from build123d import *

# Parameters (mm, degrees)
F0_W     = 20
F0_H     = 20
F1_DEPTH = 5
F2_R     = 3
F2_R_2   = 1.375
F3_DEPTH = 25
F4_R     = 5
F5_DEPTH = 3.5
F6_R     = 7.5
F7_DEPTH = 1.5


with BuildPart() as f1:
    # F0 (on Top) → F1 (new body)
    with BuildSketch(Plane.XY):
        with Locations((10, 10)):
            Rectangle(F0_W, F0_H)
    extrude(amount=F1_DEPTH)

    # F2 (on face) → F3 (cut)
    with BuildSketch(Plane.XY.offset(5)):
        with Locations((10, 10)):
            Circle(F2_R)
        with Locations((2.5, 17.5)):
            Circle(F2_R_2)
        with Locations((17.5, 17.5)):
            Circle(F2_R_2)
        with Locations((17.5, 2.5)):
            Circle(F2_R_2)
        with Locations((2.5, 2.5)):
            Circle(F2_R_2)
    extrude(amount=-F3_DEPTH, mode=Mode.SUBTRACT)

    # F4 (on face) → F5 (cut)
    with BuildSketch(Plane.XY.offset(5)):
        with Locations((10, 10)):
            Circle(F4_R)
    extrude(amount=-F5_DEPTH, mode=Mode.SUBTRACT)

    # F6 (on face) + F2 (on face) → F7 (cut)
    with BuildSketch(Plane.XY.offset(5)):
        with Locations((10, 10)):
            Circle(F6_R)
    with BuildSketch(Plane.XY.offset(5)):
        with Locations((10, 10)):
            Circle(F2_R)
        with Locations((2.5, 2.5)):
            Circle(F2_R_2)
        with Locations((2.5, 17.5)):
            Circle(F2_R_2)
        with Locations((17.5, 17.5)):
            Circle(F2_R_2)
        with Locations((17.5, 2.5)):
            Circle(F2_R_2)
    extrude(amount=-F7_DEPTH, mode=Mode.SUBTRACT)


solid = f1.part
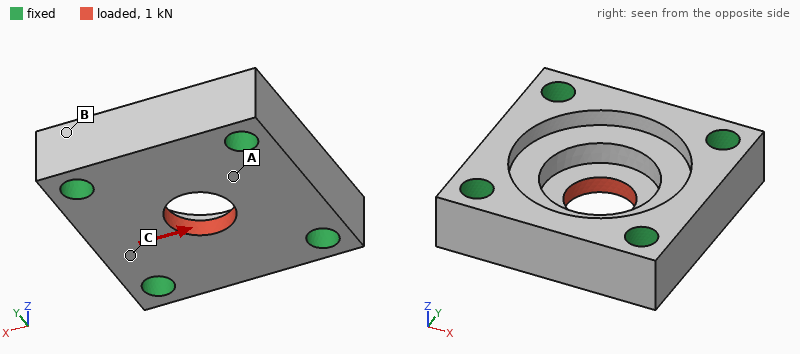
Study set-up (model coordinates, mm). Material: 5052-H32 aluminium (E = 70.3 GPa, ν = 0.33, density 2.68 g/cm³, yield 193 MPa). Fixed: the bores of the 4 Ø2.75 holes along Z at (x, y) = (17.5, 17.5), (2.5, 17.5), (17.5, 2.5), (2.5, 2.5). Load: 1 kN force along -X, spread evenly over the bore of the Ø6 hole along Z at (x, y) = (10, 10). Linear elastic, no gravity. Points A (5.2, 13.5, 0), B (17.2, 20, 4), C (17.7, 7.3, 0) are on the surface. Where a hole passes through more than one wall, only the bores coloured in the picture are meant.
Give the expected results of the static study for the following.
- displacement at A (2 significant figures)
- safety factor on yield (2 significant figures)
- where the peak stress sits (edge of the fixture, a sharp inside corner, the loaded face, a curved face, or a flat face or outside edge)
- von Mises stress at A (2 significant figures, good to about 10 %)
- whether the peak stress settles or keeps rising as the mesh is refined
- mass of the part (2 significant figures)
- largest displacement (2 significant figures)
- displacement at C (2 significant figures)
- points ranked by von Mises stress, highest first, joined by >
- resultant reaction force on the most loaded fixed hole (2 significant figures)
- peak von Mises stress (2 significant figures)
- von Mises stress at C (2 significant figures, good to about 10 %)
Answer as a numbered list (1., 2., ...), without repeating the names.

1. 1.7 µm
2. 3.0
3. the loaded face
4. 29 MPa
5. settles
6. 3.8 g
7. 4.1 µm
8. 1.7 µm
9. A > C > B
10. 270 N
11. 63 MPa
12. 17 MPa
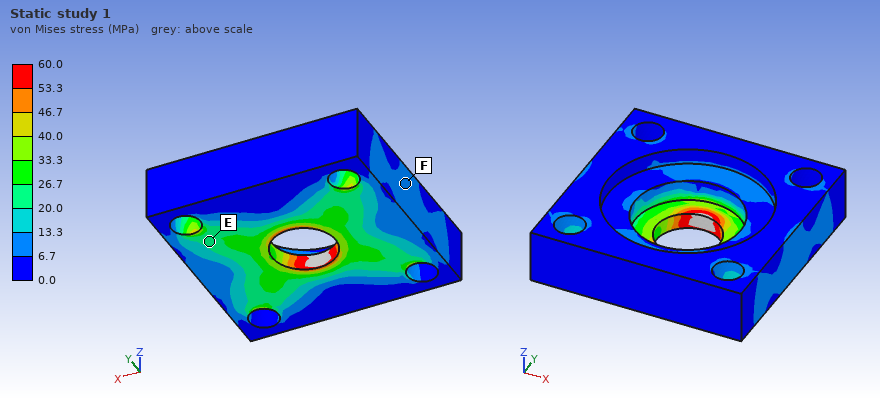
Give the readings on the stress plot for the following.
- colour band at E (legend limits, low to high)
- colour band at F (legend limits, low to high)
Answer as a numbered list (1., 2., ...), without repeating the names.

1. 20.0 to 26.7 MPa
2. 6.7 to 13.3 MPa
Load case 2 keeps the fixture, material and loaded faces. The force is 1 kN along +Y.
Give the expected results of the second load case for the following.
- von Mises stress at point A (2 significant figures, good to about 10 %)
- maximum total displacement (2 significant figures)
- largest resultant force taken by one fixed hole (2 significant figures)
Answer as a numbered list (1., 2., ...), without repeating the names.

1. 23 MPa
2. 4.1 µm
3. 270 N
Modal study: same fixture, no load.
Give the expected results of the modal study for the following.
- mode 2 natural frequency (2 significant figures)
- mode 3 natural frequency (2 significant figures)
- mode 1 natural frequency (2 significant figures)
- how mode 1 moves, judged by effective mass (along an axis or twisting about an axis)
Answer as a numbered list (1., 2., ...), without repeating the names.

1. 83 kHz
2. 88 kHz
3. 77 kHz
4. along Z
